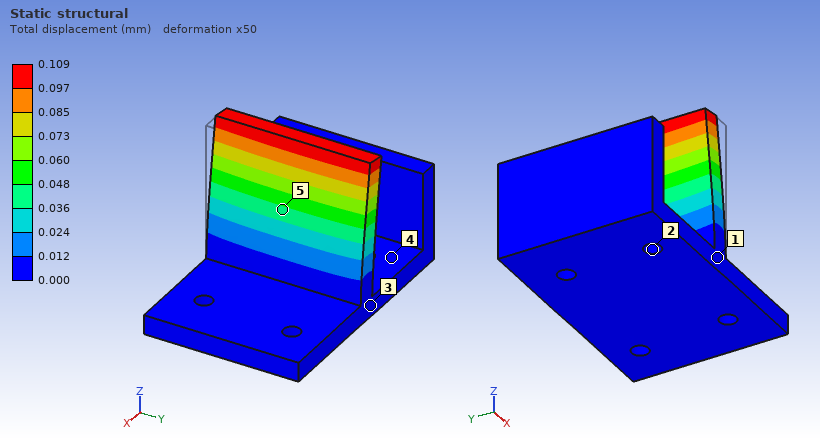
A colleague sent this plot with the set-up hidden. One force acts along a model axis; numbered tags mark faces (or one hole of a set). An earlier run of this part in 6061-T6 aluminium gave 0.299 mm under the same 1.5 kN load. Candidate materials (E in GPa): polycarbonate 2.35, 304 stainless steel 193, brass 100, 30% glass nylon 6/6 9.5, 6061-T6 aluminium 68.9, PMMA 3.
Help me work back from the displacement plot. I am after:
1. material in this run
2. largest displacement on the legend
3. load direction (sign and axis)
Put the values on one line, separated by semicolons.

304 stainless steel; 0.109 mm; -X
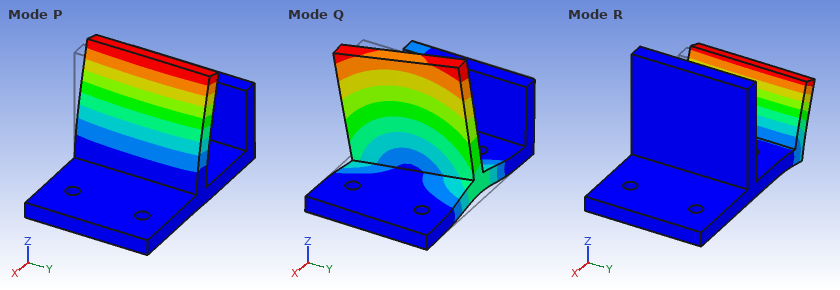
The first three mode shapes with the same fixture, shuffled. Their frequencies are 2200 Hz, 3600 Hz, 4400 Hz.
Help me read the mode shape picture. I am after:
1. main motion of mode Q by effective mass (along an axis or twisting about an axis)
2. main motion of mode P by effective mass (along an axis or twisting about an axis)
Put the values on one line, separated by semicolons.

along Y; along X
